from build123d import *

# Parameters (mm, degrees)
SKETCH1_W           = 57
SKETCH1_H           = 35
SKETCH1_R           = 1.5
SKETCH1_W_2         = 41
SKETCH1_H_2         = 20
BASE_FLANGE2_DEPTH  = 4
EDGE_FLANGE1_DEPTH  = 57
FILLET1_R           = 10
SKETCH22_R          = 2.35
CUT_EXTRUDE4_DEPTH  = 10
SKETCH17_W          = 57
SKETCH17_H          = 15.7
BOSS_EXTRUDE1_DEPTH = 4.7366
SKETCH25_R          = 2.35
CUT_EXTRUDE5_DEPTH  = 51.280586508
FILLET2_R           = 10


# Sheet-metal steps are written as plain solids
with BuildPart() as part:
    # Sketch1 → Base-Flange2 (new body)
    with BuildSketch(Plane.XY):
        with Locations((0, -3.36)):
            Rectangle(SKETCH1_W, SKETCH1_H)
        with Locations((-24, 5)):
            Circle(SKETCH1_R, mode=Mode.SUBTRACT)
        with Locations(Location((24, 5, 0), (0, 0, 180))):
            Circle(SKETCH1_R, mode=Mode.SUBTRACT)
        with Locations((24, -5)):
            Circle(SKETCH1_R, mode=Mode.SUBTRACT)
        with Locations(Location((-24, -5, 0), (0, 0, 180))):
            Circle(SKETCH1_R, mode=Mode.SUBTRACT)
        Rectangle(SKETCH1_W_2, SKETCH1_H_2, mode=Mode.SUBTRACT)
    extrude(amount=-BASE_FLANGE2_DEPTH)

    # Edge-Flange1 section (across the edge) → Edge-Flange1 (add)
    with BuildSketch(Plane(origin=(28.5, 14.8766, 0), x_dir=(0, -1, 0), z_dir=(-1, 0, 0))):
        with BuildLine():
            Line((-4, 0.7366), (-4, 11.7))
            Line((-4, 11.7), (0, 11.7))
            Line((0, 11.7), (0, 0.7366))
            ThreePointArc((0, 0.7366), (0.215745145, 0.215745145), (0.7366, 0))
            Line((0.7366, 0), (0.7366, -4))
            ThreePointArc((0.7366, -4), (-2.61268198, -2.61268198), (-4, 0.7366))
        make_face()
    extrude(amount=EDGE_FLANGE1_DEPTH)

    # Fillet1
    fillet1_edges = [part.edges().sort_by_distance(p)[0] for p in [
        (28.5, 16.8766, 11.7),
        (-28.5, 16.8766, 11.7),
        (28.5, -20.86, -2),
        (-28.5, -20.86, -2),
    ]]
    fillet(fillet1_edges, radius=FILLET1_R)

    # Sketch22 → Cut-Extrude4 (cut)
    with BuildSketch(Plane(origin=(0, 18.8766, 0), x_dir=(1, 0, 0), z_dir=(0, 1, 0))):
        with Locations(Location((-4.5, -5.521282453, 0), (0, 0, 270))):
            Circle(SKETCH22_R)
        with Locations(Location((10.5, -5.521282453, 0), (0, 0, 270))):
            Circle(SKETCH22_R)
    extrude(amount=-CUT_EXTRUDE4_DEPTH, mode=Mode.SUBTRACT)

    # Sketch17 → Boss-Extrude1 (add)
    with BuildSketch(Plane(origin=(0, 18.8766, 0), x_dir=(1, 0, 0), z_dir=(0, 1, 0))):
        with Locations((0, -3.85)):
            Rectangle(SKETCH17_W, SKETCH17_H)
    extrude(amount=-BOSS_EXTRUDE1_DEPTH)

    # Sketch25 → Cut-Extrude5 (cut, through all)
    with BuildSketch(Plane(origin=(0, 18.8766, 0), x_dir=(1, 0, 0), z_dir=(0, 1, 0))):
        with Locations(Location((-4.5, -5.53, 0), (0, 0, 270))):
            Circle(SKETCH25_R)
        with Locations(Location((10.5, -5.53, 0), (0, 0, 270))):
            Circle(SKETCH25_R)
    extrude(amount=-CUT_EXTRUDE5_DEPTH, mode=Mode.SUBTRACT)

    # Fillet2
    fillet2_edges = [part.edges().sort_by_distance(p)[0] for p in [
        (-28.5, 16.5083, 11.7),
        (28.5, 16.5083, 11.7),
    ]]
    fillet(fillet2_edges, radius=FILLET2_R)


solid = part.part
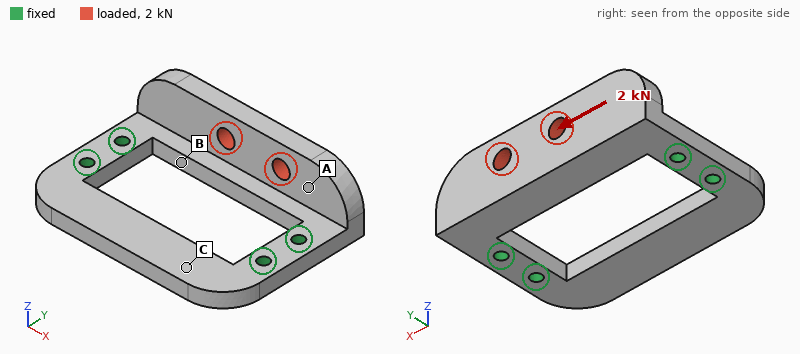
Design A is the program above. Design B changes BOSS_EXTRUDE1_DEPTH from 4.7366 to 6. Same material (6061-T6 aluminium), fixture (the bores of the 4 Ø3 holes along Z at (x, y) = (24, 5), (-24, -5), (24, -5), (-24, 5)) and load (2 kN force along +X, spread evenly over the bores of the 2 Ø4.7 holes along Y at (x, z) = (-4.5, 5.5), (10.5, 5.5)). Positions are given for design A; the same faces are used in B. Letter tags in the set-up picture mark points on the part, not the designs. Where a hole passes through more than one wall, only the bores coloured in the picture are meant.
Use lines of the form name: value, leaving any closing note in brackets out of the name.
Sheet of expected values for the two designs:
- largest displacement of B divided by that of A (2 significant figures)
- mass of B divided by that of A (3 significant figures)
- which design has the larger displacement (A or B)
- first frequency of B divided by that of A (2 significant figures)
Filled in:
largest displacement of B divided by that of A: 0.78
mass of B divided by that of A: 1.09
which design has the larger displacement: A
first frequency of B divided by that of A: 0.96
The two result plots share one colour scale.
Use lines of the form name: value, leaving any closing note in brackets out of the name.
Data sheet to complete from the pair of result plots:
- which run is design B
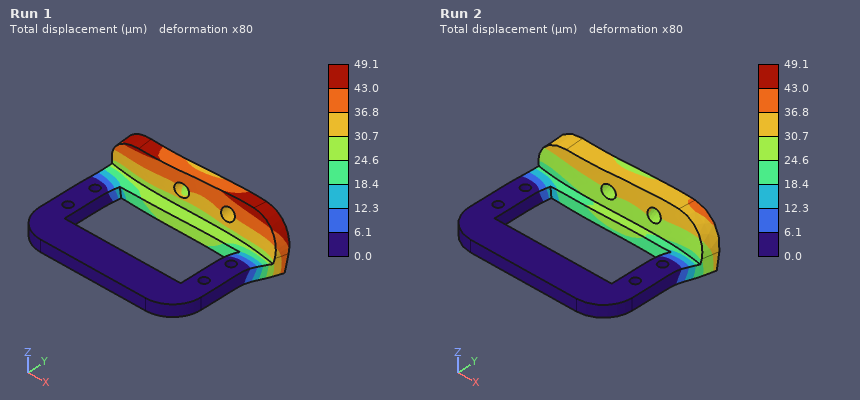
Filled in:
which run is design B: Run 2
